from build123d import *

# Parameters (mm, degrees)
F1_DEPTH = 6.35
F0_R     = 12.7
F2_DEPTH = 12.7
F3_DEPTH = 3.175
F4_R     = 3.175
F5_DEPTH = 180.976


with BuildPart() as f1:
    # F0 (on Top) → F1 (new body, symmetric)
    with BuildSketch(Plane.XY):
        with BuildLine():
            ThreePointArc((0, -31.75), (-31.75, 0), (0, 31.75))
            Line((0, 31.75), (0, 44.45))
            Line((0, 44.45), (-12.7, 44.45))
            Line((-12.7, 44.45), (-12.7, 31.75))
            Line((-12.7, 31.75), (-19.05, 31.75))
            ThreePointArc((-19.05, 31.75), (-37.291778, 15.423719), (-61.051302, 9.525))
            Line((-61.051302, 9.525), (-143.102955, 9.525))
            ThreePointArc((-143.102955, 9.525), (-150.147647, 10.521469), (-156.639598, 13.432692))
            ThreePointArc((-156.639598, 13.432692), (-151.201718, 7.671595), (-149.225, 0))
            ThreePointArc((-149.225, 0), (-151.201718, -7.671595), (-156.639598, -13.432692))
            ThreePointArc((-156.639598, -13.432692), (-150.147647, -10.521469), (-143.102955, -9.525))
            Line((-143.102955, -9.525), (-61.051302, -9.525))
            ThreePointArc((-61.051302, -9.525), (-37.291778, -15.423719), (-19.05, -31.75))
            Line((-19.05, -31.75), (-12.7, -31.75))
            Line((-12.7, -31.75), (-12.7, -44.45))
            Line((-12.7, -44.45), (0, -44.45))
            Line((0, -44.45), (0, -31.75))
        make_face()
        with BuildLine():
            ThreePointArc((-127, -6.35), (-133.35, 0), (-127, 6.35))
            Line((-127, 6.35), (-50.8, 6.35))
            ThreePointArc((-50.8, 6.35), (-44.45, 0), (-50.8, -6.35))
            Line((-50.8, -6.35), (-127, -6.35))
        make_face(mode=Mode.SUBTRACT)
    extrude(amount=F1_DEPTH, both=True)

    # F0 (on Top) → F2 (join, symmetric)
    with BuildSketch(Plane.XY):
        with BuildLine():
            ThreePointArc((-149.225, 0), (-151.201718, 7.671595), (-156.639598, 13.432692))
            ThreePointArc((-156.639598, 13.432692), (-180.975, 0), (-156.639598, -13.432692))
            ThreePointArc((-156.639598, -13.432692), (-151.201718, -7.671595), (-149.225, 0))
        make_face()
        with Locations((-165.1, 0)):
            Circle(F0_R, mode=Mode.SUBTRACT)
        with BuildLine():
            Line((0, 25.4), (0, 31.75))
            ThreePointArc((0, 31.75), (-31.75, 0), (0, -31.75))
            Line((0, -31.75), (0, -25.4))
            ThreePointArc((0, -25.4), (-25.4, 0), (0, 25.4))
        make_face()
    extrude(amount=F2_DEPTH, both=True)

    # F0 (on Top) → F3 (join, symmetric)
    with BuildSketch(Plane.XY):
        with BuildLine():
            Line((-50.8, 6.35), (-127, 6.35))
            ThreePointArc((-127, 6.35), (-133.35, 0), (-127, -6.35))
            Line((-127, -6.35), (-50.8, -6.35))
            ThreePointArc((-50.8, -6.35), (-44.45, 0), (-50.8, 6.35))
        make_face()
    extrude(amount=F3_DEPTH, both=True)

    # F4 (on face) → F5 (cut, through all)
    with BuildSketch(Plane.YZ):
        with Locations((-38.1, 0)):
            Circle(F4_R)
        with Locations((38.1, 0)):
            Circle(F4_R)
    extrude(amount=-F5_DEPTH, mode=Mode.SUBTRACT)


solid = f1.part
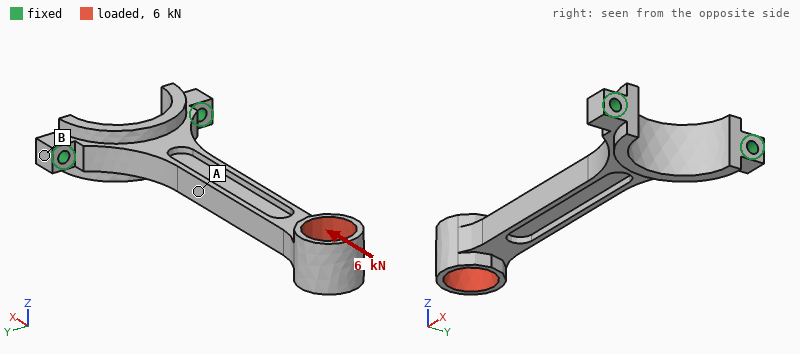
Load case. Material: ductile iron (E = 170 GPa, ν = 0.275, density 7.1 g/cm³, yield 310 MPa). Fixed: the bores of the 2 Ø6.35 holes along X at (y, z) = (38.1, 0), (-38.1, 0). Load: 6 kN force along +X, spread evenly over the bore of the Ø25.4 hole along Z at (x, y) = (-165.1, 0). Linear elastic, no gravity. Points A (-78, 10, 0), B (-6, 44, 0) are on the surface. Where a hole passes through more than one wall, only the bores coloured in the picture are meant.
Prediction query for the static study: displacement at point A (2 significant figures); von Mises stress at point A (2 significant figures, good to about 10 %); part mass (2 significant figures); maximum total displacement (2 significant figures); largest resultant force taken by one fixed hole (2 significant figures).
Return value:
16 µm
37 MPa
370 g
66 µm
3.8 kN
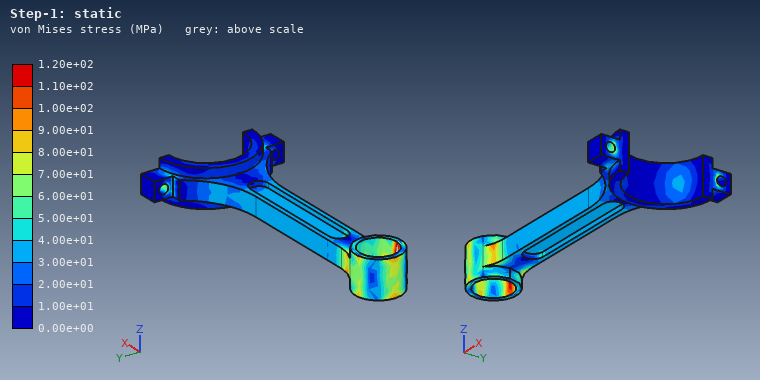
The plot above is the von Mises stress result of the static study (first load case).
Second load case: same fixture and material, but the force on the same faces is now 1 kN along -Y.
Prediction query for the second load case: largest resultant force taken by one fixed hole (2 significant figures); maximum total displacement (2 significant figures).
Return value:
2.9 kN
0.82 mm
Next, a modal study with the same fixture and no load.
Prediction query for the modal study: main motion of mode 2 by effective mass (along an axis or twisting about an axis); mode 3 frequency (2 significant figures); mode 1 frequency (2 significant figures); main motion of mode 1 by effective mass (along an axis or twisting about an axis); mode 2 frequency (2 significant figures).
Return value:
along Y
1700 Hz
300 Hz
along Z
680 Hz
